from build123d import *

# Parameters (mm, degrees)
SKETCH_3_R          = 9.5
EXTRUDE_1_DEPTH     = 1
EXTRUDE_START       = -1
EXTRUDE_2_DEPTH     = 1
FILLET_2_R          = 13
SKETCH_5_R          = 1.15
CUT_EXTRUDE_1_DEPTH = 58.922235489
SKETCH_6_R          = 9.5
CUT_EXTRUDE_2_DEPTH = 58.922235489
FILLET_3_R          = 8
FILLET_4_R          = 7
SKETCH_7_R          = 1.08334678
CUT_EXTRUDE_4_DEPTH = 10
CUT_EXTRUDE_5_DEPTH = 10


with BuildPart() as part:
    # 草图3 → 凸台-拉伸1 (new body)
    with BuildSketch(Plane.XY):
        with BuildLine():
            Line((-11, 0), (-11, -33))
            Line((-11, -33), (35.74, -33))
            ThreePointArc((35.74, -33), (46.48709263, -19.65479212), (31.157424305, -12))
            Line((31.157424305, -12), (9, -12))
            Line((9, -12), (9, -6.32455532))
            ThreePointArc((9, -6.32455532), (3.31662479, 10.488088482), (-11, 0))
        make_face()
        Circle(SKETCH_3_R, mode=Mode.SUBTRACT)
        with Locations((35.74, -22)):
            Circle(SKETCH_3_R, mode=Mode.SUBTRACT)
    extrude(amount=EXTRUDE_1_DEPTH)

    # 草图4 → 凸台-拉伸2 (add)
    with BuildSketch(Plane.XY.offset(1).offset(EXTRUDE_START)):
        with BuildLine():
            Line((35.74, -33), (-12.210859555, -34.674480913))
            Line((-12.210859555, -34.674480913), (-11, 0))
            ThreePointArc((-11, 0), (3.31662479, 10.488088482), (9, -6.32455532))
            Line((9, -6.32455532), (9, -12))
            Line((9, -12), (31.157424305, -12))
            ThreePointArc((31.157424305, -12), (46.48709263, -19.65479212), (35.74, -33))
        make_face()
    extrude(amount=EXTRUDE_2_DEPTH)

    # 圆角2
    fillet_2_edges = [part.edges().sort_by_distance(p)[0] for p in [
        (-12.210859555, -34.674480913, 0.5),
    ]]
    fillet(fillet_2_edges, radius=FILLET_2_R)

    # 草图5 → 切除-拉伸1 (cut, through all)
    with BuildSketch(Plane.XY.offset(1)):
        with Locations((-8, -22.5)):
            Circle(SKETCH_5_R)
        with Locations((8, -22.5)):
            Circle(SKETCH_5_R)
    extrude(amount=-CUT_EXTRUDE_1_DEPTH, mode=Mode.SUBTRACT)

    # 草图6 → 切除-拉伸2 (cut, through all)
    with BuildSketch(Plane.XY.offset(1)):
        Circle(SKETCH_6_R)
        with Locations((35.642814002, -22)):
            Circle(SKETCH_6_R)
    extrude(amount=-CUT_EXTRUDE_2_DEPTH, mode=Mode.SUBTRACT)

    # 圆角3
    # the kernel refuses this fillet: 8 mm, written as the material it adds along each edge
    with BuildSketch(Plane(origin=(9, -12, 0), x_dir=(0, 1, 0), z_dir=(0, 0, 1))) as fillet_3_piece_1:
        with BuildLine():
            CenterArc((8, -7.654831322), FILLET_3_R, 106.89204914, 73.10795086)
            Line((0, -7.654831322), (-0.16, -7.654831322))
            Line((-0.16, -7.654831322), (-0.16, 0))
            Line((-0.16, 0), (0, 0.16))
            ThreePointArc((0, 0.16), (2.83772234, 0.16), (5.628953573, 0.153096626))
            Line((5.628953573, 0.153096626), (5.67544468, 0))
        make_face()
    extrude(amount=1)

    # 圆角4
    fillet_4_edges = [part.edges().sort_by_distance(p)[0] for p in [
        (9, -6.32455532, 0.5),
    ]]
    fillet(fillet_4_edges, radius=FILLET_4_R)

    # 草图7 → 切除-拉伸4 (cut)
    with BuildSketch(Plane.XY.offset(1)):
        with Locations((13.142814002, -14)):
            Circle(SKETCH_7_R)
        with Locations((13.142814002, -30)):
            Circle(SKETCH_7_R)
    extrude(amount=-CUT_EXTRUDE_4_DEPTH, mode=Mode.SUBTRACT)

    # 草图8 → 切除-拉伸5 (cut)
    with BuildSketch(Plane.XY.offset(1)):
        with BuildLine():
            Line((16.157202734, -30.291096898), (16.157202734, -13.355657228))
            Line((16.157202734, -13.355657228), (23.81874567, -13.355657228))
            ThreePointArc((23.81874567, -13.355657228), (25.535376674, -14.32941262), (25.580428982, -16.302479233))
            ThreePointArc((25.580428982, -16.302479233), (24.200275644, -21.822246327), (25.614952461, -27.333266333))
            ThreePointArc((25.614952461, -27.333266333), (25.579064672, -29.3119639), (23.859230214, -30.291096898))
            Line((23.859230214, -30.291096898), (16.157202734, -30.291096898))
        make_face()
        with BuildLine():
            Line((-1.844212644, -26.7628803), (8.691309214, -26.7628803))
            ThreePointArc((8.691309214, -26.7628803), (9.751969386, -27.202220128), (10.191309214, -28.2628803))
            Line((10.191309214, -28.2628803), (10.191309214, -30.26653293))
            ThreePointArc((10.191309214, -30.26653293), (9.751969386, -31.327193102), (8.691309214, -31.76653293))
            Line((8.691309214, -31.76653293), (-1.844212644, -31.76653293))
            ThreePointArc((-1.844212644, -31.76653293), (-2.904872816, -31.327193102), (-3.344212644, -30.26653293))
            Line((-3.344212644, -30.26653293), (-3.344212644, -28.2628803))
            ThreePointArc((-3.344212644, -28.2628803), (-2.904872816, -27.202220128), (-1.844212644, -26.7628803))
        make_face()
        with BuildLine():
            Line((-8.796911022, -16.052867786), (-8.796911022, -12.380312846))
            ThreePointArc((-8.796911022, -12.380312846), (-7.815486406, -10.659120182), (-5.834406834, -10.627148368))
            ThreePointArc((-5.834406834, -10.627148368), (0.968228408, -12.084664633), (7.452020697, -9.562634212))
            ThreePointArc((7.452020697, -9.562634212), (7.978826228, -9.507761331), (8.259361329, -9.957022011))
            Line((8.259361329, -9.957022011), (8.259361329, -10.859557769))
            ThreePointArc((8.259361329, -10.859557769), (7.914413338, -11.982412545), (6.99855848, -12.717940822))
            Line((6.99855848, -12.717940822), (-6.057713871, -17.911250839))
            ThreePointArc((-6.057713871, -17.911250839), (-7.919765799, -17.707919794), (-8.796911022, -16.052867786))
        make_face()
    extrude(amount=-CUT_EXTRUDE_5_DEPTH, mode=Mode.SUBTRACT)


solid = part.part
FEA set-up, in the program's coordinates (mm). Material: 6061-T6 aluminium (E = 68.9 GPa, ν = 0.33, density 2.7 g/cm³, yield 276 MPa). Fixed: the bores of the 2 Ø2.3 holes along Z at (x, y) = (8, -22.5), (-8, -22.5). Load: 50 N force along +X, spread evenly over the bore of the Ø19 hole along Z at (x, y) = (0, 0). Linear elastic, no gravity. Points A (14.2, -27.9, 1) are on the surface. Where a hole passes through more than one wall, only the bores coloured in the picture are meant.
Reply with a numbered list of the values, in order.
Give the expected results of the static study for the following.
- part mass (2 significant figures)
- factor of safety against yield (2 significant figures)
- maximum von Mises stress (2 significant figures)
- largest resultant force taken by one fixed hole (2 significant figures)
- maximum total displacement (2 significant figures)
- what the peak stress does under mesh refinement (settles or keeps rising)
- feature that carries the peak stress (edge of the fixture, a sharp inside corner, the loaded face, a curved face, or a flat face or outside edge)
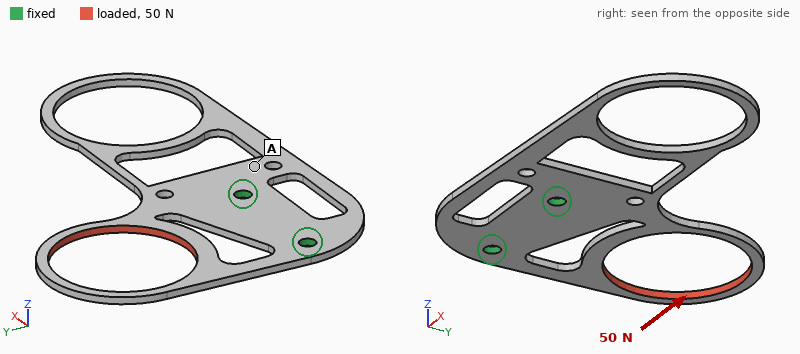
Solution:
1. 2.1 g
2. 1.4
3. 200 MPa
4. 67 N
5. 0.15 mm
6. settles
7. a curved face
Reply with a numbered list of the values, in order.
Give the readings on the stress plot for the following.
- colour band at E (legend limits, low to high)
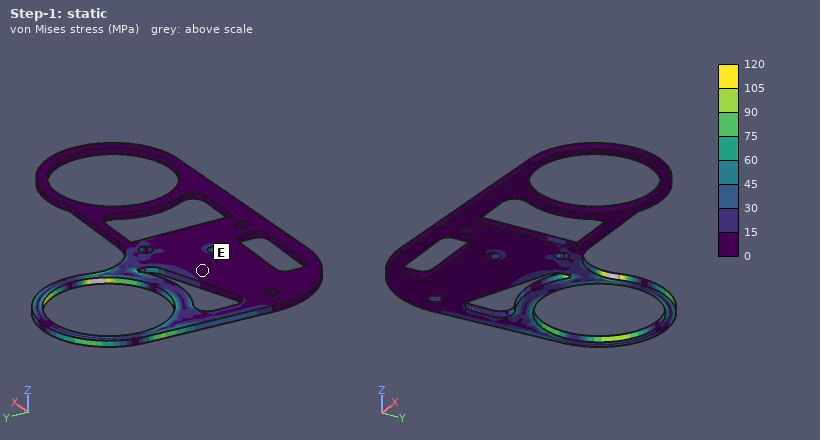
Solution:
1. 0 to 15 MPa
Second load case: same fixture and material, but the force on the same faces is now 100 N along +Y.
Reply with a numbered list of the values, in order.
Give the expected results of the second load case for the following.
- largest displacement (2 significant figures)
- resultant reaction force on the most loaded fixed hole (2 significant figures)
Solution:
1. 35 µm
2. 51 N
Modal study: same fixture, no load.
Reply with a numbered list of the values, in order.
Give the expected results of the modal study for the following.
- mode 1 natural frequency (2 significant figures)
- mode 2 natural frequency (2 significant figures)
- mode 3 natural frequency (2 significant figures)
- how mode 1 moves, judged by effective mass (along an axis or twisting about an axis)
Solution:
1. 630 Hz
2. 1000 Hz
3. 1700 Hz
4. along Z
